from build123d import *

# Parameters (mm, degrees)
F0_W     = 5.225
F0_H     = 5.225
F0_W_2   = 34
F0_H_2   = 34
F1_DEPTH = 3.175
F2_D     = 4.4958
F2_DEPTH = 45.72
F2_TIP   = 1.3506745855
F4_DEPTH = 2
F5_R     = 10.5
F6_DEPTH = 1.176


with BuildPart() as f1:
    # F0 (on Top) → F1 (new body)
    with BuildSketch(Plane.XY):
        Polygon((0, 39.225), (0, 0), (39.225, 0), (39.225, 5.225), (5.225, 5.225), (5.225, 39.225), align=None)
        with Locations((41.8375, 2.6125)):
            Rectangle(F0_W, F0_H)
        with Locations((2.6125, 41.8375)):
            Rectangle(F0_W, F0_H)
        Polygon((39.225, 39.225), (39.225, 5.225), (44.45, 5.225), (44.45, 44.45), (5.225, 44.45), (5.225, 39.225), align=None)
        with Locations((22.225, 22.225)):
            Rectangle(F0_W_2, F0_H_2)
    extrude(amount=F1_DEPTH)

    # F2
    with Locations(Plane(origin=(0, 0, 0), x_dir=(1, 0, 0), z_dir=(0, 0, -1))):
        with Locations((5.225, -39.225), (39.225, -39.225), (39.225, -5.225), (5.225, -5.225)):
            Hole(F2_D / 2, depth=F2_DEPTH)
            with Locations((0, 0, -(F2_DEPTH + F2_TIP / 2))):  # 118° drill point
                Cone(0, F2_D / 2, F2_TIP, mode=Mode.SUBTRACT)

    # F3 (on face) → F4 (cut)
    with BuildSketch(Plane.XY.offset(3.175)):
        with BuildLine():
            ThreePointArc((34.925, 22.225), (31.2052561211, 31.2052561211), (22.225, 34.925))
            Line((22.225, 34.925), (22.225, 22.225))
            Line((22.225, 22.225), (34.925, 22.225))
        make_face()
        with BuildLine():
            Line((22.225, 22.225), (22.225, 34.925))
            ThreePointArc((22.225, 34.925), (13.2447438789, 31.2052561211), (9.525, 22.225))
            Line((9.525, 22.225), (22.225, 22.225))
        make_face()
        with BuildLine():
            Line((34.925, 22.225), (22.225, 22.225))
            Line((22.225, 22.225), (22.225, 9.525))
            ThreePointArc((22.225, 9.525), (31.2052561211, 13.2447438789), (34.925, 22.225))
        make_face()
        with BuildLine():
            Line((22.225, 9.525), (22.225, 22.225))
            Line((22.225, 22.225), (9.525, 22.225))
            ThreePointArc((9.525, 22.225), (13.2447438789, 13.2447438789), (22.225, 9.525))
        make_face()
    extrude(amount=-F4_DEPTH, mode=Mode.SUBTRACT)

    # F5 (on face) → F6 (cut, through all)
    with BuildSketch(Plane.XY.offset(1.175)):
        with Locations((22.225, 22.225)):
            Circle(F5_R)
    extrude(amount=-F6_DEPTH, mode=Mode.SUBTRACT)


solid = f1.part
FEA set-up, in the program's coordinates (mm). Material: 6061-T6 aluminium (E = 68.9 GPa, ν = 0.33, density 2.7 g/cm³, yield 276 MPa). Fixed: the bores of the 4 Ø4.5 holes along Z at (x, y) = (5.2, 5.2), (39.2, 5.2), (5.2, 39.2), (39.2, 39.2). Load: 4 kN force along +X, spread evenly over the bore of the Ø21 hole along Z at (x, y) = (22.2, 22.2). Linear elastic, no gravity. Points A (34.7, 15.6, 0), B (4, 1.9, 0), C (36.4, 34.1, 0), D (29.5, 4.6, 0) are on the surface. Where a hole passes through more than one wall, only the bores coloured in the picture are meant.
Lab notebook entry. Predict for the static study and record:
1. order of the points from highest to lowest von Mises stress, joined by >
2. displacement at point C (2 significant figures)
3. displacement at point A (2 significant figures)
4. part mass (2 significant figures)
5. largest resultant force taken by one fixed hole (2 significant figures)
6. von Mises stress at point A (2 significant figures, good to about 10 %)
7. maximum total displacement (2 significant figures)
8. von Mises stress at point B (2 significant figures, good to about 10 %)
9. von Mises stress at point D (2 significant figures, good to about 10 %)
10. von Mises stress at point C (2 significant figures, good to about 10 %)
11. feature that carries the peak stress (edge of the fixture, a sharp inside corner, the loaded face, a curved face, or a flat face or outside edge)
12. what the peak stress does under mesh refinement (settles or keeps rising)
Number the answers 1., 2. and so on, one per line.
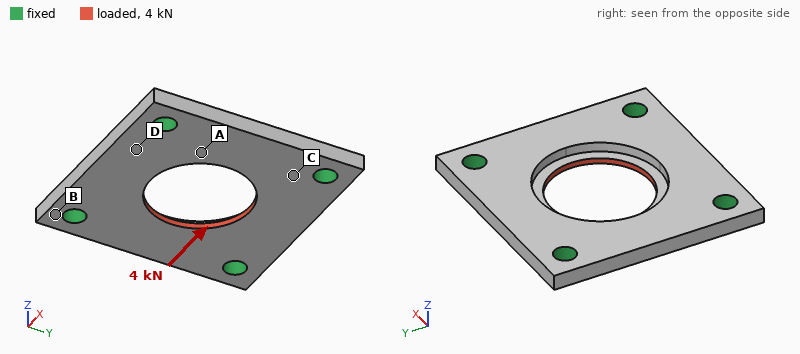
1. A > C > D > B
2. 4.3 µm
3. 11 µm
4. 13 g
5. 1.1 kN
6. 56 MPa
7. 22 µm
8. 7.5 MPa
9. 16 MPa
10. 44 MPa
11. edge of the fixture
12. keeps rising
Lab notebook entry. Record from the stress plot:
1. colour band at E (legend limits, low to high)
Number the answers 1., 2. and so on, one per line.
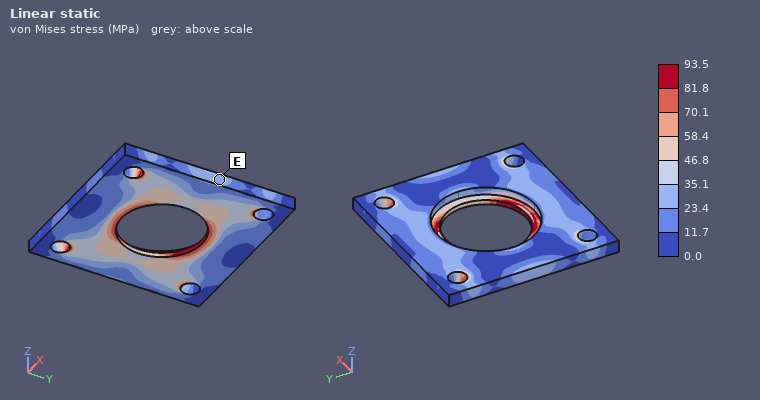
1. 23.4 to 35.1 MPa
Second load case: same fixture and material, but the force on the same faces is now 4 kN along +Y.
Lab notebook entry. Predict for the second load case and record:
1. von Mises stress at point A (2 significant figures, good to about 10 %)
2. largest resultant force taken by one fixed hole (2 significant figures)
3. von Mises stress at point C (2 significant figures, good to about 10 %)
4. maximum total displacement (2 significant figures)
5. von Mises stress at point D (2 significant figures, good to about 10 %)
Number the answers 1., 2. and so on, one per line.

1. 34 MPa
2. 1.1 kN
3. 36 MPa
4. 22 µm
5. 37 MPa
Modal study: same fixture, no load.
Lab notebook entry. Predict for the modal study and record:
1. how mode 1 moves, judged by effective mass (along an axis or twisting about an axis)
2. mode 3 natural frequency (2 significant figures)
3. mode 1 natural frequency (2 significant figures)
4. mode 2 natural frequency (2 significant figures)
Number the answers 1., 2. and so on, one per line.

1. along Z
2. 16 kHz
3. 15 kHz
4. 16 kHz
